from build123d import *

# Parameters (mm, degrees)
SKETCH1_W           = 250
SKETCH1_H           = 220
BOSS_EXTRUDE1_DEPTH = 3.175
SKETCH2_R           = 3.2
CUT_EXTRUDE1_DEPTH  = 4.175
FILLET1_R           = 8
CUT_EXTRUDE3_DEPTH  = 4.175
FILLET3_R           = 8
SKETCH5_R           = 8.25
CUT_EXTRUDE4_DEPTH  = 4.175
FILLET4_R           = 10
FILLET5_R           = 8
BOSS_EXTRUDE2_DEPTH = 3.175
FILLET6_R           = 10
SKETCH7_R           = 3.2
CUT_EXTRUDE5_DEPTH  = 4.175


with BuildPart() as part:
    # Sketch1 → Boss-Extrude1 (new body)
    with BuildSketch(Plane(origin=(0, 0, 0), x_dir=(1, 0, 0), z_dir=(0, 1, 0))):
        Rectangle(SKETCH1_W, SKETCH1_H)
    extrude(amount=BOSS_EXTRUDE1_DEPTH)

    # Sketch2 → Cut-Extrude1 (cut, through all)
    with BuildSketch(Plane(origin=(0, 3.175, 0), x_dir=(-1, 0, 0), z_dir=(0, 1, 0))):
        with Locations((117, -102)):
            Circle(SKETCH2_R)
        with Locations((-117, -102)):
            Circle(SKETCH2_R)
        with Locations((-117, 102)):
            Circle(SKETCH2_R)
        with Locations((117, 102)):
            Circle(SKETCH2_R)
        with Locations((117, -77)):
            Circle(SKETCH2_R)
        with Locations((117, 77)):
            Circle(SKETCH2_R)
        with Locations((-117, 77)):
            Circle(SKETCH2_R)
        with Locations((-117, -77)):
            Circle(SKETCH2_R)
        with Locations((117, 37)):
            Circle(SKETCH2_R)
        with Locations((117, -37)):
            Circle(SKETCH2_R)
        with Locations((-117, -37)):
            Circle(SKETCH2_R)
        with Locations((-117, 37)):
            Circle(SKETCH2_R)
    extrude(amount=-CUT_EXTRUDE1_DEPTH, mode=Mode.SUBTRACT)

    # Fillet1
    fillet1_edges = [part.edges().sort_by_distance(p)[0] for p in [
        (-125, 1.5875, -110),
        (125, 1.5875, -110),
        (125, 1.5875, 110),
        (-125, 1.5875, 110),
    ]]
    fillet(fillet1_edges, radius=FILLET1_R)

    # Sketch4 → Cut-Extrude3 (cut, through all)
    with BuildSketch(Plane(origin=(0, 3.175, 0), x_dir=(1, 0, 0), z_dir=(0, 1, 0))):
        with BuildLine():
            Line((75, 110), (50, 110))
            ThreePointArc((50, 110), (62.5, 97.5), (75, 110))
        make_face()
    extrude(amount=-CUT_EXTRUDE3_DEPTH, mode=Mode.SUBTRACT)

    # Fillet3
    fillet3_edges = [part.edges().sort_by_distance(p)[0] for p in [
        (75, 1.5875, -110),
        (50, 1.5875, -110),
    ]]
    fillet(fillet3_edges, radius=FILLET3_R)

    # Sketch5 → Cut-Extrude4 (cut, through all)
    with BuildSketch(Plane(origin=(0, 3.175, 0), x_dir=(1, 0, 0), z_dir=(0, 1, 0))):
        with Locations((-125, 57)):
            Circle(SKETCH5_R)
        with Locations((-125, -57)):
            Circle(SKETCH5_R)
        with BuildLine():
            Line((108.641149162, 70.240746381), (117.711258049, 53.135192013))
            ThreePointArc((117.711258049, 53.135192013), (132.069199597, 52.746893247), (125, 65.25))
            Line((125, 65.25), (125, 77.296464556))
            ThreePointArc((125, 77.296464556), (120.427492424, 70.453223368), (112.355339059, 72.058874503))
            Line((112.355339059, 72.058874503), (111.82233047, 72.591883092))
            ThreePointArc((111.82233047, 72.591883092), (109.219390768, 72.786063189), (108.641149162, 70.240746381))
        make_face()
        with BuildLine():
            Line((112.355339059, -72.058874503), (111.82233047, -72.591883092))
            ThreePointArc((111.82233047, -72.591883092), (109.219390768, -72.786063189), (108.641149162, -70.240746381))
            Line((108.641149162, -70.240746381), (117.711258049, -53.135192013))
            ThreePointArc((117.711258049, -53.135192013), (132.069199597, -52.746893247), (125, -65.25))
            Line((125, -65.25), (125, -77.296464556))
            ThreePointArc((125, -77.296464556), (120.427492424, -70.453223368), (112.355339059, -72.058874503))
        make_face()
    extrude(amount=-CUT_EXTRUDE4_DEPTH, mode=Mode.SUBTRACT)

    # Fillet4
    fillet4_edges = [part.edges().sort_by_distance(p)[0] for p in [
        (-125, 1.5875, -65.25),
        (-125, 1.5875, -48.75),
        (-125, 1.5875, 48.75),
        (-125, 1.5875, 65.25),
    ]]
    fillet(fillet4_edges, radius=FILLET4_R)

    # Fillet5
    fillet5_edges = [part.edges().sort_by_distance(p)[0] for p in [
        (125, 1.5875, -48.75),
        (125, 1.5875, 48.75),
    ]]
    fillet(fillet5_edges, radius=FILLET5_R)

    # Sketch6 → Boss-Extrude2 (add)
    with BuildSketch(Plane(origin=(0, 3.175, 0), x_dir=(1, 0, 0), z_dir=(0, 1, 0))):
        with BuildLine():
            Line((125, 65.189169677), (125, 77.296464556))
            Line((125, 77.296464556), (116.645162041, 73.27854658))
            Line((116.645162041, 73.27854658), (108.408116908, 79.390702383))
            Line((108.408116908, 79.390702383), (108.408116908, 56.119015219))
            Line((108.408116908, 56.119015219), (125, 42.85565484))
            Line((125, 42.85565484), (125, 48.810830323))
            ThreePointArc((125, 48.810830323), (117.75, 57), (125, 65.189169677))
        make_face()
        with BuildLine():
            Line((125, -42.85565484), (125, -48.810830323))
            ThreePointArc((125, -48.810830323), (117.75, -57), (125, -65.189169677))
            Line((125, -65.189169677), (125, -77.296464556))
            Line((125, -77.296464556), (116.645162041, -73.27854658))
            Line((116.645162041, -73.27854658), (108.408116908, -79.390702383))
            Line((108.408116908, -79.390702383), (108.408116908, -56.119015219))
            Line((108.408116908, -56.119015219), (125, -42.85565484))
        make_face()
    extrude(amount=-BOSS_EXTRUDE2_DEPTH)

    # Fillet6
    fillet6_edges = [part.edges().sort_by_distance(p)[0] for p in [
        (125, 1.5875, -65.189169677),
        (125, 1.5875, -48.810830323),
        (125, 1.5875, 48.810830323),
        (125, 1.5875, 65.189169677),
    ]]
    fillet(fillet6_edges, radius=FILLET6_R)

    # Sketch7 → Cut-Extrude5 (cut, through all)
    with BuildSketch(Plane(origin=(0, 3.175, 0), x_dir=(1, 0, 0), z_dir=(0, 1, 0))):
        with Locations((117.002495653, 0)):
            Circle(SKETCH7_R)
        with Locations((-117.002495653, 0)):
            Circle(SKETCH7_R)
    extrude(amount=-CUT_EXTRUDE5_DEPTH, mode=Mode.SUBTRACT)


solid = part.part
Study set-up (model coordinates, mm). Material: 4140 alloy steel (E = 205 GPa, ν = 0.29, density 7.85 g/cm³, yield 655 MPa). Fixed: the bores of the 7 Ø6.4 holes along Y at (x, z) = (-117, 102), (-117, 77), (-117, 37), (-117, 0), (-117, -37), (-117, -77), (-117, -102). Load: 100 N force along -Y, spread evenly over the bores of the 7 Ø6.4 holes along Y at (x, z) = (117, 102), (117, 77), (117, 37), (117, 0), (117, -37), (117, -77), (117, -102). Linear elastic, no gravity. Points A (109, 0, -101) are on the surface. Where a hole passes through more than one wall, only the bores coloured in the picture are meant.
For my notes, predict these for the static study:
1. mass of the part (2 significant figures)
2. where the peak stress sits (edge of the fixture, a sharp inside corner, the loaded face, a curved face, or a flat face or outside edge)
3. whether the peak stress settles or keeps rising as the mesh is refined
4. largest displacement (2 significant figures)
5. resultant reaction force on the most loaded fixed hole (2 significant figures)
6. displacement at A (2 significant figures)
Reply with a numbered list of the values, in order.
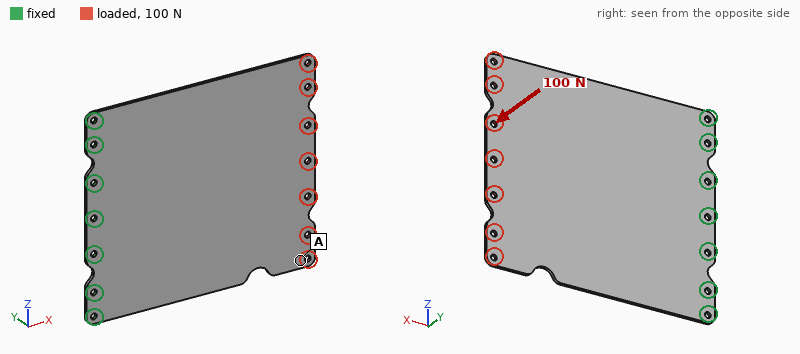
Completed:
1. 1.3 kg
2. edge of the fixture
3. keeps rising
4. 3.6 mm
5. 43 N
6. 3.2 mm
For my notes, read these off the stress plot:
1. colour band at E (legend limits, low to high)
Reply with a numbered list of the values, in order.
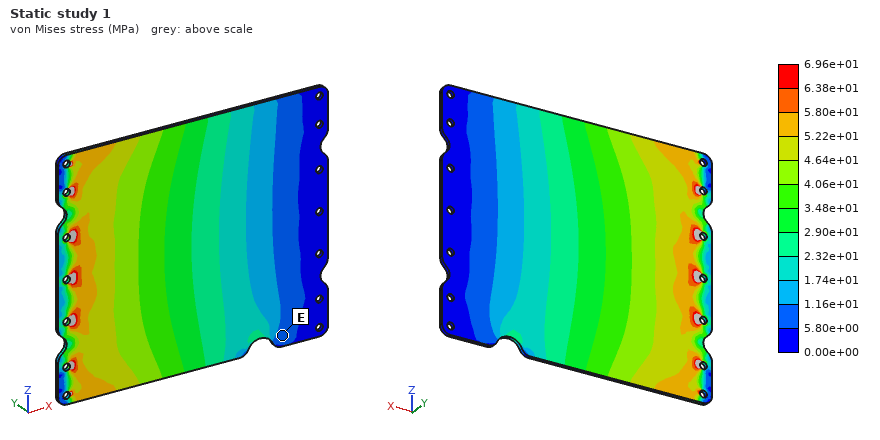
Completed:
1. 5.80e+00 to 1.16e+01 MPa
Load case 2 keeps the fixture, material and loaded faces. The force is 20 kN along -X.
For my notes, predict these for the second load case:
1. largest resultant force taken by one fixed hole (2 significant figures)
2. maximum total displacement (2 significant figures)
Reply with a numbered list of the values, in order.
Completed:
1. 3.2 kN
2. 49 µm
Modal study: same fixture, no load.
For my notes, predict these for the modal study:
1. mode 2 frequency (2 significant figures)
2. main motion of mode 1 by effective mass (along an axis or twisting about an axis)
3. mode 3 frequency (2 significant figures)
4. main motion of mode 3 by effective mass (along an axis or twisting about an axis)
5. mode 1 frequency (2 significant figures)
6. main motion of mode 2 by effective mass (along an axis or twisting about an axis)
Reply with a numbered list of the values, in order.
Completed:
1. 120 Hz
2. along Y
3. 290 Hz
4. along Y
5. 47 Hz
6. twisting about X
